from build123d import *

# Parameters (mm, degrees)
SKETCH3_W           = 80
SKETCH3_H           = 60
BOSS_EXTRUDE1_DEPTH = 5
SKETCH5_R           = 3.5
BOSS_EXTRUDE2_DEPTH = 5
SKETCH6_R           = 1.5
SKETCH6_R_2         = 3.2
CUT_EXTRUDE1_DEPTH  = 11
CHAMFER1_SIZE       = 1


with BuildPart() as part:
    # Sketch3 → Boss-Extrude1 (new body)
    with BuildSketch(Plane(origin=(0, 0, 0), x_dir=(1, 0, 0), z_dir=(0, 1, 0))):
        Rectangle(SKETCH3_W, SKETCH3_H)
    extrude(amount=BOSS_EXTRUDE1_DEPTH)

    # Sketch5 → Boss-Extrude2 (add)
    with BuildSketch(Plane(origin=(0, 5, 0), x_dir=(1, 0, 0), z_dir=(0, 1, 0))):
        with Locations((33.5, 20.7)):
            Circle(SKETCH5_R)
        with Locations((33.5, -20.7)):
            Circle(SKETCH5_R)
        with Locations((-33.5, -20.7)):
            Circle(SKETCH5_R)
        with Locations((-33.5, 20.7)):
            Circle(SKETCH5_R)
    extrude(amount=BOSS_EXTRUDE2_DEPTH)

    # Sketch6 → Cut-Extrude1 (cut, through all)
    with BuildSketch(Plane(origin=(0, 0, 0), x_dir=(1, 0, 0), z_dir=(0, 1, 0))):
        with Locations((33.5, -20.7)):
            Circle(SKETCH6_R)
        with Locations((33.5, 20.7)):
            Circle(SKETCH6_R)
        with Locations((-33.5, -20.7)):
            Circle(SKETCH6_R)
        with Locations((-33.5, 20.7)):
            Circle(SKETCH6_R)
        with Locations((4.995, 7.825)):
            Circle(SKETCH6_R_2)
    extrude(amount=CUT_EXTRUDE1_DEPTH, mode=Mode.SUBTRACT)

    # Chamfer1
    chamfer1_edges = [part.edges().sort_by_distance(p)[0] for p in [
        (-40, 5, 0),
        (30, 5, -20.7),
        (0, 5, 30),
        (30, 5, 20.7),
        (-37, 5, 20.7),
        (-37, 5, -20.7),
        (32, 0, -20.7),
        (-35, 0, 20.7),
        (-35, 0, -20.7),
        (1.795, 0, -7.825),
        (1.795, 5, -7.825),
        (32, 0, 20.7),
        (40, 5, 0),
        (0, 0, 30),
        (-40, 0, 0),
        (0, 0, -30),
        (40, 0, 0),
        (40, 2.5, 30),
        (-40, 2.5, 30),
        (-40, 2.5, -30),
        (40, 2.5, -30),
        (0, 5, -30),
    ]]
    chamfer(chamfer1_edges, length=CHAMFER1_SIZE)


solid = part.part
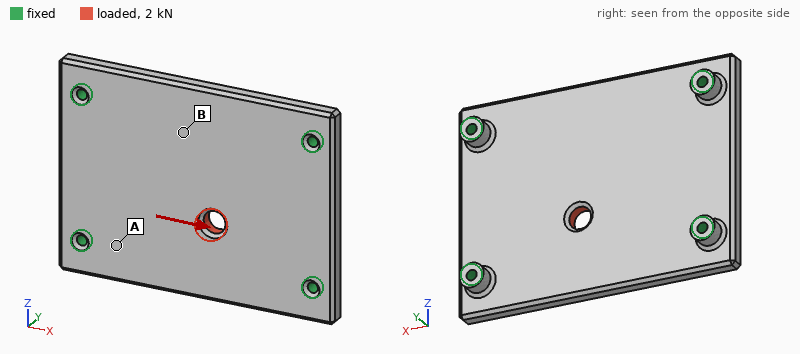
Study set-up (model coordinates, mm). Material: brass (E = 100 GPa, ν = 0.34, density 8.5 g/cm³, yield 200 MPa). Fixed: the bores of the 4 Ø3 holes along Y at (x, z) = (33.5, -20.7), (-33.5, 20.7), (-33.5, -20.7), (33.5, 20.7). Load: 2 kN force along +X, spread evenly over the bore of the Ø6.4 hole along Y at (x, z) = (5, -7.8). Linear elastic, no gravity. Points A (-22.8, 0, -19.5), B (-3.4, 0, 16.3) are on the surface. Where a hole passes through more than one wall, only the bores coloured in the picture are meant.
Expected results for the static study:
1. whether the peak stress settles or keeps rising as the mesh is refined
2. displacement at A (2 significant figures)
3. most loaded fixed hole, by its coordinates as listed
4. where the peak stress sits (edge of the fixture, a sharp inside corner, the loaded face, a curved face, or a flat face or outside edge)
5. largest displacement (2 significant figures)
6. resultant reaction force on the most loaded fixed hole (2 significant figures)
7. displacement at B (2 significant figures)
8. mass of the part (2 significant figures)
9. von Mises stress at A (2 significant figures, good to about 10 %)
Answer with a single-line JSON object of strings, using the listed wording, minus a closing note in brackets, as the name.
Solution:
{"whether the peak stress settles or keeps rising as the mesh is refined": "keeps rising", "displacement at A": "0.99 µm", "most loaded fixed hole, by its coordinates as listed": "(33.5, -20.7)", "where the peak stress sits": "edge of the fixture", "largest displacement": "3.8 µm", "resultant reaction force on the most loaded fixed hole": "700 N", "displacement at B": "0.90 µm", "mass of the part": "200 g", "von Mises stress at A": "6.1 MPa"}
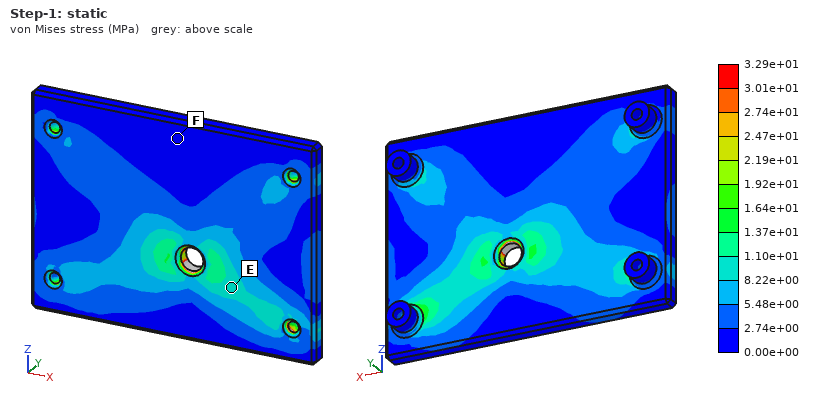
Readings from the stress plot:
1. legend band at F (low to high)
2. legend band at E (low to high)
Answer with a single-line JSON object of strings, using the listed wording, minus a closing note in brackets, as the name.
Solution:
{"legend band at F": "0.00e+00 to 2.74e+00 MPa", "legend band at E": "8.22e+00 to 1.10e+01 MPa"}
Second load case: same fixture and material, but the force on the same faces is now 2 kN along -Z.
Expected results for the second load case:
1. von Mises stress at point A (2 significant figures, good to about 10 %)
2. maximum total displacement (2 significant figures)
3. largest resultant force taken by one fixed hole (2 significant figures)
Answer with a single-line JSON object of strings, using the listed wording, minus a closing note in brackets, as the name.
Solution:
{"von Mises stress at point A": "4.3 MPa", "maximum total displacement": "5.9 µm", "largest resultant force taken by one fixed hole": "670 N"}
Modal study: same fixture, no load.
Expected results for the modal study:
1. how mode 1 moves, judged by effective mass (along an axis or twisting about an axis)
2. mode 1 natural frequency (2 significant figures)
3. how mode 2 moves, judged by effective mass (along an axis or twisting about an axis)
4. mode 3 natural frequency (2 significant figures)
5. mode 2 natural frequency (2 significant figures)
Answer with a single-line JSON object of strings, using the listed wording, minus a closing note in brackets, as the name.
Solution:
{"how mode 1 moves, judged by effective mass": "along Y", "mode 1 natural frequency": "3400 Hz", "how mode 2 moves, judged by effective mass": "twisting about X", "mode 3 natural frequency": "7200 Hz", "mode 2 natural frequency": "4600 Hz"}
